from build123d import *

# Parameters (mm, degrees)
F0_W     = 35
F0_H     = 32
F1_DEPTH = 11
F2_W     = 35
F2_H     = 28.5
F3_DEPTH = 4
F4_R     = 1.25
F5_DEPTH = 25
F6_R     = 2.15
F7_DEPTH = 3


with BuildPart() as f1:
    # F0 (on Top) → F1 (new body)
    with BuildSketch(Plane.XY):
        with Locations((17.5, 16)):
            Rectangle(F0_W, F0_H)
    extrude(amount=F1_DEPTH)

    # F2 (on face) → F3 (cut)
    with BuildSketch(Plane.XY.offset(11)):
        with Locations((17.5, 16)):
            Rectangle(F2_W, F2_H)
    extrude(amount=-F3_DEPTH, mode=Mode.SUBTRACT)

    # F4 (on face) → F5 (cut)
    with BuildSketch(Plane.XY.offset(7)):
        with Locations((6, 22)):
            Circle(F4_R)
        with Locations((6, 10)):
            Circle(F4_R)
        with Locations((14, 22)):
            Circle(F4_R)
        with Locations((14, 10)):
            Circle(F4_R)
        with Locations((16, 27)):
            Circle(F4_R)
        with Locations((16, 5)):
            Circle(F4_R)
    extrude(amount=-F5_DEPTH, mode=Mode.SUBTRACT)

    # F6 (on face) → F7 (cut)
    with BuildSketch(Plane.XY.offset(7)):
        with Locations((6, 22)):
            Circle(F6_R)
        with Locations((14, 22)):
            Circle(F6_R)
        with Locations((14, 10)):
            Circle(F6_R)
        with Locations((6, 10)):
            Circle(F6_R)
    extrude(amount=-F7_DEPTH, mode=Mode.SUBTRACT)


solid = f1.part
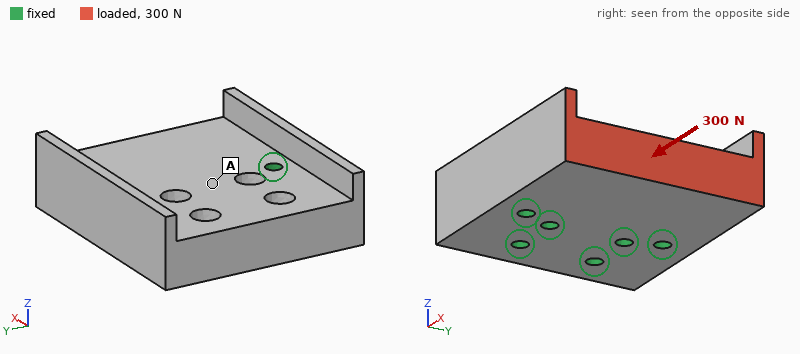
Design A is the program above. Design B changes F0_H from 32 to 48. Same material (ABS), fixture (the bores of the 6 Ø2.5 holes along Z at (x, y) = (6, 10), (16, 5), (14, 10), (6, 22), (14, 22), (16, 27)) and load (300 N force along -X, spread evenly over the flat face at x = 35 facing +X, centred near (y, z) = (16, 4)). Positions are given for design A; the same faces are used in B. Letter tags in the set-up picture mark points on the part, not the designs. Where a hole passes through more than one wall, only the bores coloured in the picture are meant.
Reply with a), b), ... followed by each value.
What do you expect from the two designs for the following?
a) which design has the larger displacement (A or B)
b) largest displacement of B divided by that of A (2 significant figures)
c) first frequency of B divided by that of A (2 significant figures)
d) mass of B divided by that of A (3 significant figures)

a) B
b) 1.2
c) 0.86
d) 1.77
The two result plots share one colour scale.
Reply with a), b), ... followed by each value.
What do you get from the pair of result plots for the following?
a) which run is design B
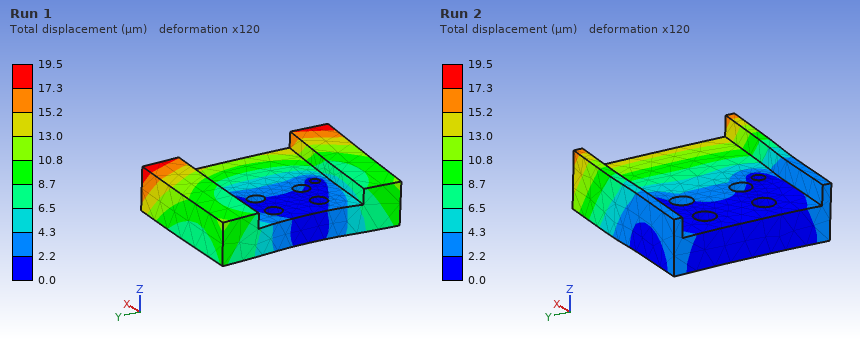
a) Run 1
